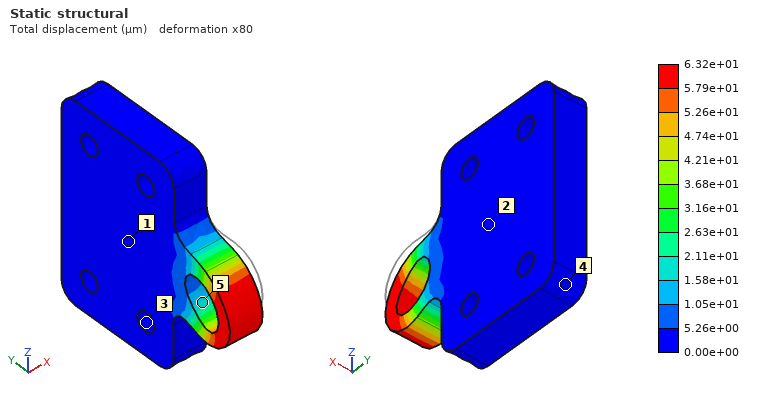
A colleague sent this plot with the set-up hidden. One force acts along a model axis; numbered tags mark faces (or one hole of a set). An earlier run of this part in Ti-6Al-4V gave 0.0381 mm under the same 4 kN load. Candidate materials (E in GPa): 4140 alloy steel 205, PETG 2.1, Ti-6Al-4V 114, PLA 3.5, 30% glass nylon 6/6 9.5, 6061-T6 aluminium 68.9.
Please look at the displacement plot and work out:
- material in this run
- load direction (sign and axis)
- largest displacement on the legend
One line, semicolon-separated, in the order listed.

6061-T6 aluminium; -Z; 6.32e+01 µm
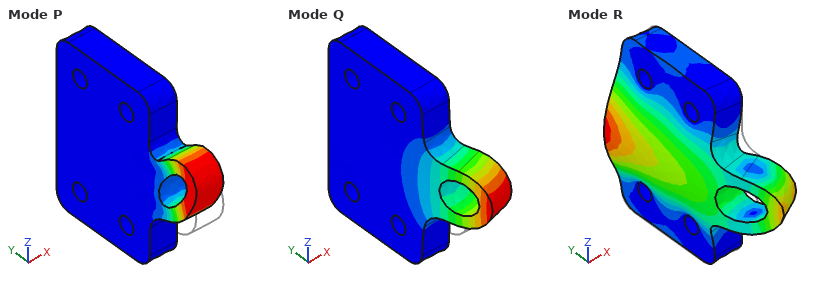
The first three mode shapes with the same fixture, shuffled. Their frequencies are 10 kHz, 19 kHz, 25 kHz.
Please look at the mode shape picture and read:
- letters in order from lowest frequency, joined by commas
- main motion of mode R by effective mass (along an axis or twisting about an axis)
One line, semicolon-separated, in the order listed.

Q, P, R; along X
